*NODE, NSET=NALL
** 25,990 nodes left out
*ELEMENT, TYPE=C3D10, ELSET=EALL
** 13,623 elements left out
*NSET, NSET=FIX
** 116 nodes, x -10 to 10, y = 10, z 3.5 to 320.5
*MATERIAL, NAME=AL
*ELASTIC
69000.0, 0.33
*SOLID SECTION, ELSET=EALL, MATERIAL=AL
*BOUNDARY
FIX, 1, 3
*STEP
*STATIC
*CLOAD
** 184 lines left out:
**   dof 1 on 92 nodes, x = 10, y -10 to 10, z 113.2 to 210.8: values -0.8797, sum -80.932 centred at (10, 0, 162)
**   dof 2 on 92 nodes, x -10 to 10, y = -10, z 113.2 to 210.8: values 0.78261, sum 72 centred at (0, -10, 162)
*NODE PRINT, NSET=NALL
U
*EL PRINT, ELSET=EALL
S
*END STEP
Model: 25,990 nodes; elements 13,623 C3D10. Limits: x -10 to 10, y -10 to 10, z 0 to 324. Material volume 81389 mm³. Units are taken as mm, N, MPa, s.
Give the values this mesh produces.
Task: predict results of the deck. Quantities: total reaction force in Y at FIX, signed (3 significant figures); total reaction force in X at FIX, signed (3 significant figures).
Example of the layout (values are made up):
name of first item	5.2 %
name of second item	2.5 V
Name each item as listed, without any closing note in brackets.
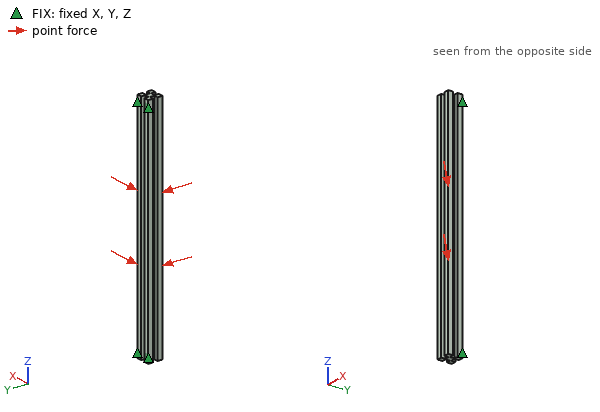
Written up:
total reaction force in Y at FIX, signed	-72.0 N
total reaction force in X at FIX, signed	80.9 N
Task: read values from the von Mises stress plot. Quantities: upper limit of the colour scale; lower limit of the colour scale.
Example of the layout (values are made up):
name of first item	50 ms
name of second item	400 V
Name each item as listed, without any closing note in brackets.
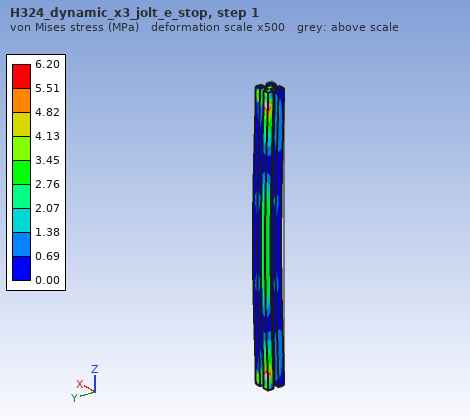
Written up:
upper limit of the colour scale	6.20 MPa
lower limit of the colour scale	0.00 MPa
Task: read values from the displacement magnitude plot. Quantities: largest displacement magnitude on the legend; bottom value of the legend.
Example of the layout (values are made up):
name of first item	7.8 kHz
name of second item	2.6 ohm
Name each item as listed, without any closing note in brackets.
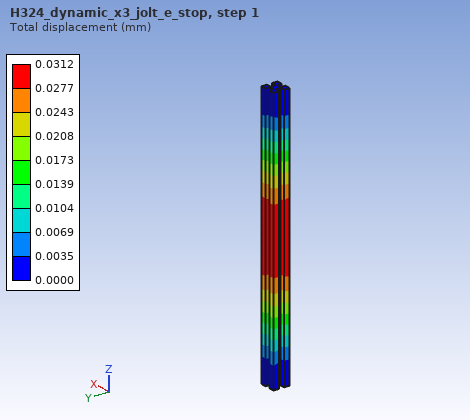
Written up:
largest displacement magnitude on the legend	0.0312 mm
bottom value of the legend	0.0000 mm
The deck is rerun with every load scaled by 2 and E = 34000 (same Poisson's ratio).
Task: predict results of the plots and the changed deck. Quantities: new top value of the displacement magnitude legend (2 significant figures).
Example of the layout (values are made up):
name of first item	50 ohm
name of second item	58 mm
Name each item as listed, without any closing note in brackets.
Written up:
new top value of the displacement magnitude legend	0.13 mm
